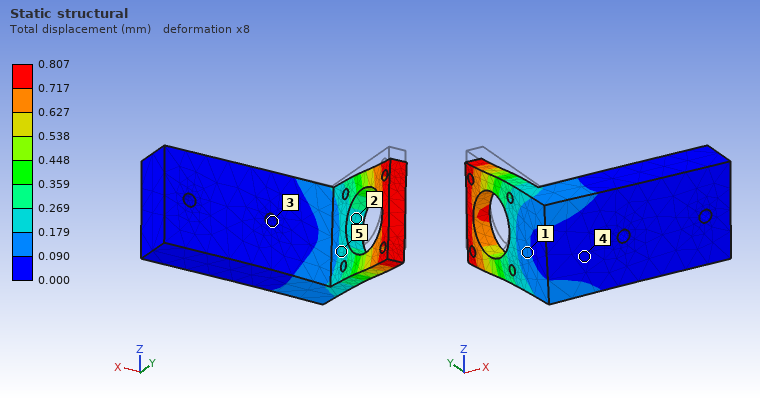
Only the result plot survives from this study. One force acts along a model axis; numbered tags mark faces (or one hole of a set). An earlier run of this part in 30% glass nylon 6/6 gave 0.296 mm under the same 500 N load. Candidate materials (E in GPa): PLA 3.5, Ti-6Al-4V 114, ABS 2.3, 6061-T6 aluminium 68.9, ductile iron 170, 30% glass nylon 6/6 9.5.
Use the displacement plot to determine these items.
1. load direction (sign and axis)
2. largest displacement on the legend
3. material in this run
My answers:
-Z
0.807 mm
PLA
